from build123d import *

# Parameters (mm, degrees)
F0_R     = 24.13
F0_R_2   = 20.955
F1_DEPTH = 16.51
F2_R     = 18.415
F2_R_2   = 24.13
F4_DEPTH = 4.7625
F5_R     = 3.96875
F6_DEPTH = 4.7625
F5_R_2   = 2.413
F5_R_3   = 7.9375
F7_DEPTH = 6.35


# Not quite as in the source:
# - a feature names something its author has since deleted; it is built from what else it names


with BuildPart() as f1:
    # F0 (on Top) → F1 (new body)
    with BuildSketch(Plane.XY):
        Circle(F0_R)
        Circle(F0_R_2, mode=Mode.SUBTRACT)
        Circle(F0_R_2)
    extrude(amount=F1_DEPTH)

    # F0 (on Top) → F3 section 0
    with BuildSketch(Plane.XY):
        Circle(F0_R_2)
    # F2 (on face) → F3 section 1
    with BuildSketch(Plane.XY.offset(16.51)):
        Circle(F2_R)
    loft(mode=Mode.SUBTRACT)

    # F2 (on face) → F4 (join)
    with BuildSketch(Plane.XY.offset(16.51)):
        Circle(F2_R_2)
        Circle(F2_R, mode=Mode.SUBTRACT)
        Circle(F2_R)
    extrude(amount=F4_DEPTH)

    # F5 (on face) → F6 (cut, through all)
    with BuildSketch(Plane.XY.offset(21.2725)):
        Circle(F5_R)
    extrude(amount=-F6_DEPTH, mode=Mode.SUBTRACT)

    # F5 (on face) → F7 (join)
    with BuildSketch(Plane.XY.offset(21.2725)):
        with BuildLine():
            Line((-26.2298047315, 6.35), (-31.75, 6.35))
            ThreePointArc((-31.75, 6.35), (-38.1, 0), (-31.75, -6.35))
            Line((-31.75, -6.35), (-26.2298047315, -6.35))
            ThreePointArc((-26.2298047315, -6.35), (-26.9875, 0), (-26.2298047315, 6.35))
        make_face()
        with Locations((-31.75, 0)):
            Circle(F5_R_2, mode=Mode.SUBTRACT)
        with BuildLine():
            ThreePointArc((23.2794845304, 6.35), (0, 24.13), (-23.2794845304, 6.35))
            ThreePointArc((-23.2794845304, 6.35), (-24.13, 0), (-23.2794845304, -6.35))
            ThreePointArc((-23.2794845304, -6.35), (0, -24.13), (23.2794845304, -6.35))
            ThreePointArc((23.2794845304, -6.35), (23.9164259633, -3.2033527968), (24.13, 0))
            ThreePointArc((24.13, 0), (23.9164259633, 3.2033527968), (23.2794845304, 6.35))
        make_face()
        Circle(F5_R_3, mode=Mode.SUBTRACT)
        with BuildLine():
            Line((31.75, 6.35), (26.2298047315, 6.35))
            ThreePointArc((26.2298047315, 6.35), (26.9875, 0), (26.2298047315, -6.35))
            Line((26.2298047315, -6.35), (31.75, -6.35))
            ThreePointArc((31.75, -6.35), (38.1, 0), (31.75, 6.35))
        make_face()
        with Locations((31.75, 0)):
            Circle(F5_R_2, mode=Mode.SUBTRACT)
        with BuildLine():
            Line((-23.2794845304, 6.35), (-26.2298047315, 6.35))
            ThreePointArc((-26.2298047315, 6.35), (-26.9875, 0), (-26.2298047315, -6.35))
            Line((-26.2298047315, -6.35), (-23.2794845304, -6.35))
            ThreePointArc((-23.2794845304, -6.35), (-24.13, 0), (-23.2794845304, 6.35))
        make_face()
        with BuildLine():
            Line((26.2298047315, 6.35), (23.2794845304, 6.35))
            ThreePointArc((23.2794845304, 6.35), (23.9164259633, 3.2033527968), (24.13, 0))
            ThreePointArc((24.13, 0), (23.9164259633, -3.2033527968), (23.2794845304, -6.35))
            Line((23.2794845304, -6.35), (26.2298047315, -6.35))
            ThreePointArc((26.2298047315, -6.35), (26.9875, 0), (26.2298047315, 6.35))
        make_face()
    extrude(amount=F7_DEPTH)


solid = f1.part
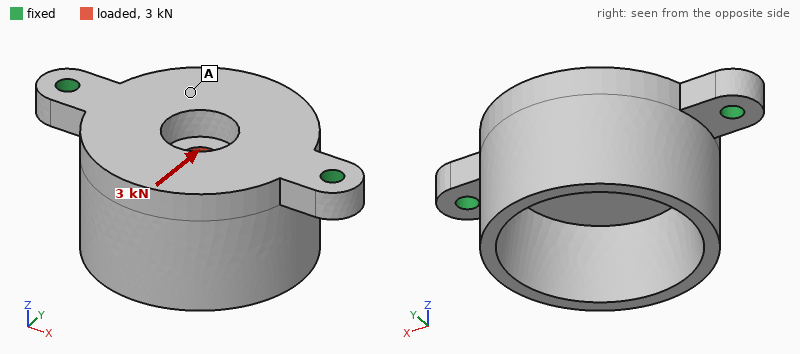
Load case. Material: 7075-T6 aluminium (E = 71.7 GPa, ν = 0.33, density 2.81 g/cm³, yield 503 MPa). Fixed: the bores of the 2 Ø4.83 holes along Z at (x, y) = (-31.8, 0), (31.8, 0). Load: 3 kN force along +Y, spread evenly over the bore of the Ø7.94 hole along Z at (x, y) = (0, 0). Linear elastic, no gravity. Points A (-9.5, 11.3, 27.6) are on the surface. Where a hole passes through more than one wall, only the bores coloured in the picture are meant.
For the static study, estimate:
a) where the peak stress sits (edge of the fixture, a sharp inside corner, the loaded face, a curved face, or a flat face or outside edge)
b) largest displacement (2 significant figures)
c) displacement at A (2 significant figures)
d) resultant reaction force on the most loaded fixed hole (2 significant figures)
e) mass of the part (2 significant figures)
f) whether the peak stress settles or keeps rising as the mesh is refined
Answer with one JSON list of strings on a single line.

["edge of the fixture", "0.12 mm", "0.037 mm", "1.5 kN", "86 g", "keeps rising"]
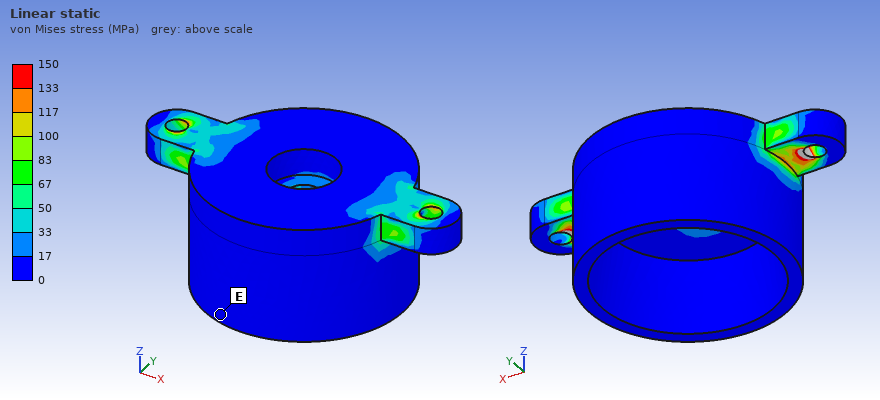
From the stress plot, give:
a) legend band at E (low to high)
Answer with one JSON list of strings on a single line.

["0 to 17 MPa"]
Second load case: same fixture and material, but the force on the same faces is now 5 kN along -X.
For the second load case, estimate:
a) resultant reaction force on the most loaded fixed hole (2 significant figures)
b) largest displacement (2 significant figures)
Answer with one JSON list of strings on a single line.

["2.6 kN", "12 µm"]
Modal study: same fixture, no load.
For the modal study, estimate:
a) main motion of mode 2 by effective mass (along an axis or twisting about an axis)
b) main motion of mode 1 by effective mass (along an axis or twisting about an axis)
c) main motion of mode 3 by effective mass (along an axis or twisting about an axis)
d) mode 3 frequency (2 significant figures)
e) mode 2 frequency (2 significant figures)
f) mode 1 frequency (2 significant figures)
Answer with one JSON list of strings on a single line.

["along Z", "along Y", "along Y", "9900 Hz", "6100 Hz", "2300 Hz"]
